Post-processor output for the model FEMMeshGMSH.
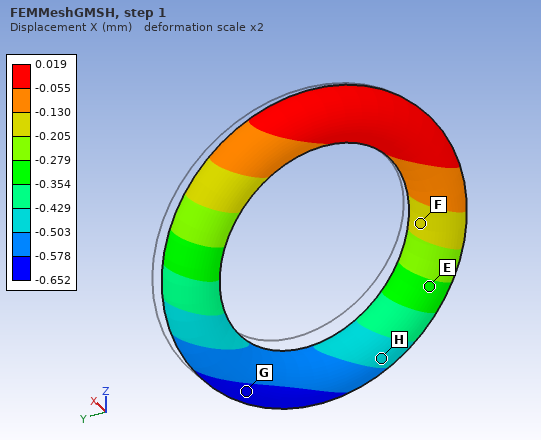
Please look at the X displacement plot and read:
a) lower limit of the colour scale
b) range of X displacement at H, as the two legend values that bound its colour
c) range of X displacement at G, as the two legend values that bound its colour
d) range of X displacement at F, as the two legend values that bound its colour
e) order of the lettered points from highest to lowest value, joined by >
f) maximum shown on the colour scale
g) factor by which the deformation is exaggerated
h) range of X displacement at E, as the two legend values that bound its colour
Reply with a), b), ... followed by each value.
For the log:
a) -0.652 mm
b) -0.503 to -0.429 mm
c) -0.652 to -0.578 mm
d) -0.205 to -0.130 mm
e) F > E > H > G
f) 0.019 mm
g) 2
h) -0.354 to -0.279 mm
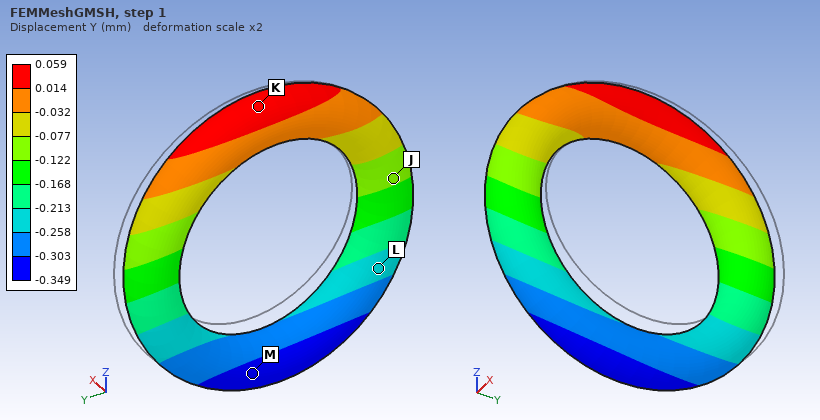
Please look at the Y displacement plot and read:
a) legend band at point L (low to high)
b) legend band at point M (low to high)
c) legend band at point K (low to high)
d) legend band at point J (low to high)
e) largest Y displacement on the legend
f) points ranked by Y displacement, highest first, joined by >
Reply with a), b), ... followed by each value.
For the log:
a) -0.258 to -0.213 mm
b) -0.349 to -0.303 mm
c) 0.014 to 0.059 mm
d) -0.122 to -0.077 mm
e) 0.059 mm
f) K > J > L > M
